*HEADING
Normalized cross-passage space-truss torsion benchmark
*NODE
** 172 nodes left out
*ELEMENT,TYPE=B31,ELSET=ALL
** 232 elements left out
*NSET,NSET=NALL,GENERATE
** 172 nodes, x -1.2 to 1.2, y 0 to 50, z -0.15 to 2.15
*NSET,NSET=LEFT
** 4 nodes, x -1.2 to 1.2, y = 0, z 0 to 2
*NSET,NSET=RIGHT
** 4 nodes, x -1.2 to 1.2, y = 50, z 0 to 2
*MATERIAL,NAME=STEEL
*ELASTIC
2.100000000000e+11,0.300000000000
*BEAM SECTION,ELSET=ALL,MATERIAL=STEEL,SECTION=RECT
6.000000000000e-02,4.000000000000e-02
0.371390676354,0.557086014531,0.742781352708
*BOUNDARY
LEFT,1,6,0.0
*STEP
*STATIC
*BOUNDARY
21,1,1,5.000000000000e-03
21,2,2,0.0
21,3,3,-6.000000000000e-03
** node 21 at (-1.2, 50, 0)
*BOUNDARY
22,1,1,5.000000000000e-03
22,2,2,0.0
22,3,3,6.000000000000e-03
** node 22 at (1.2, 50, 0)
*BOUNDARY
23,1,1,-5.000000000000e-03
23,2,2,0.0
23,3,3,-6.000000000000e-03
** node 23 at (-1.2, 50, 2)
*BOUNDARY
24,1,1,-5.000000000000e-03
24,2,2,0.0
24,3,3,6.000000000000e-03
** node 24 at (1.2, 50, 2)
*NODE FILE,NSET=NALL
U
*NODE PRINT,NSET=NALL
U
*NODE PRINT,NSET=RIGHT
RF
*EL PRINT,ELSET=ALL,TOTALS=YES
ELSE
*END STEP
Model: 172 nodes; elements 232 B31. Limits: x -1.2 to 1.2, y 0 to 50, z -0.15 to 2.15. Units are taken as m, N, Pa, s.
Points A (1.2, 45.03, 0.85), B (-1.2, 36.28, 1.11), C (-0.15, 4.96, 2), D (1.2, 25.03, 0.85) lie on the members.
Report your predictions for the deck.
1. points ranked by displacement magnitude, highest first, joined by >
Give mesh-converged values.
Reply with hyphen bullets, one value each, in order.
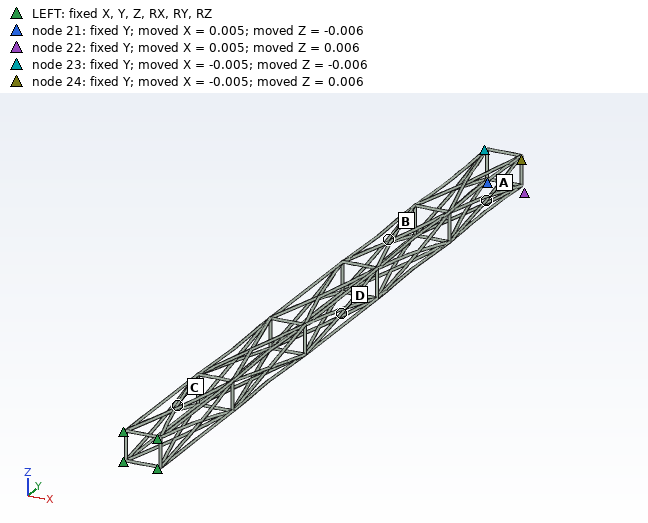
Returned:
- A > B > D > C
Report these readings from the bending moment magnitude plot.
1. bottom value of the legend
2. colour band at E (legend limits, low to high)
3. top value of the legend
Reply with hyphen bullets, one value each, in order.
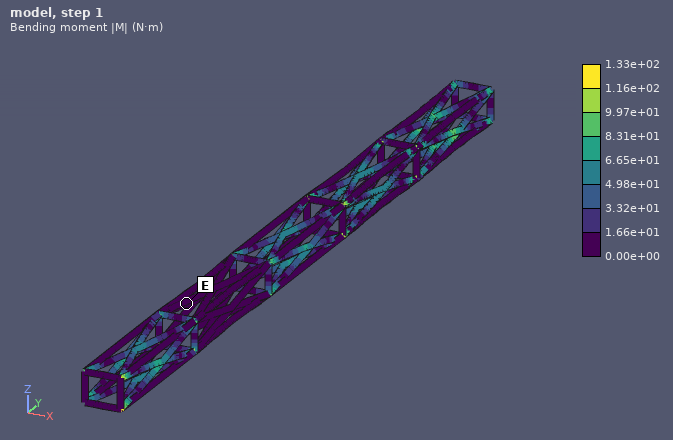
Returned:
- 0.00e+00 N·m
- 0.00e+00 to 1.66e+01 N·m
- 1.33e+02 N·m
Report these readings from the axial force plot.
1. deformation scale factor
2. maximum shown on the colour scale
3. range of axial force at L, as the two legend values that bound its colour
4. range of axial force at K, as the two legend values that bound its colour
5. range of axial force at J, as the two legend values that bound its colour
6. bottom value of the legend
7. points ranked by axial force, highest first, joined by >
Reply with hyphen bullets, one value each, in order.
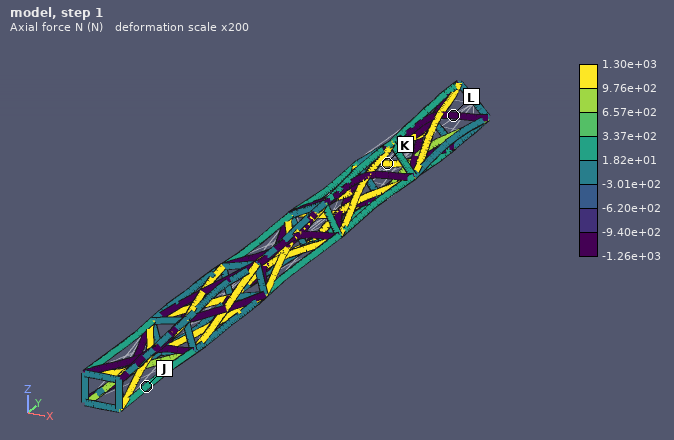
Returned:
- 200
- 1.30e+03 N
- -1.26e+03 to -9.40e+02 N
- 9.76e+02 to 1.30e+03 N
- 1.82e+01 to 3.37e+02 N
- -1.26e+03 N
- K > J > L
